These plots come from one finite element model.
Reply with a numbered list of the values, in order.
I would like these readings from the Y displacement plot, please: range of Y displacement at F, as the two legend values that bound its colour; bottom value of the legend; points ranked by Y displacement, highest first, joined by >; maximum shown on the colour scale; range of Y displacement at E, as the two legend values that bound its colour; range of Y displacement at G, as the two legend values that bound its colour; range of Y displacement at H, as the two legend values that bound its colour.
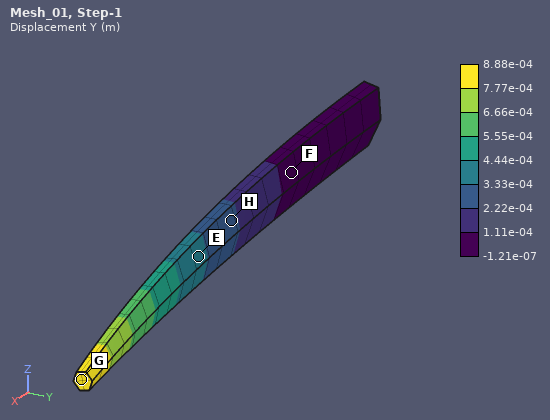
1. -1.21e-07 to 1.11e-04 m
2. -1.21e-07 m
3. G > E > H > F
4. 8.88e-04 m
5. 3.33e-04 to 4.44e-04 m
6. 7.77e-04 to 8.88e-04 m
7. 2.22e-04 to 3.33e-04 m
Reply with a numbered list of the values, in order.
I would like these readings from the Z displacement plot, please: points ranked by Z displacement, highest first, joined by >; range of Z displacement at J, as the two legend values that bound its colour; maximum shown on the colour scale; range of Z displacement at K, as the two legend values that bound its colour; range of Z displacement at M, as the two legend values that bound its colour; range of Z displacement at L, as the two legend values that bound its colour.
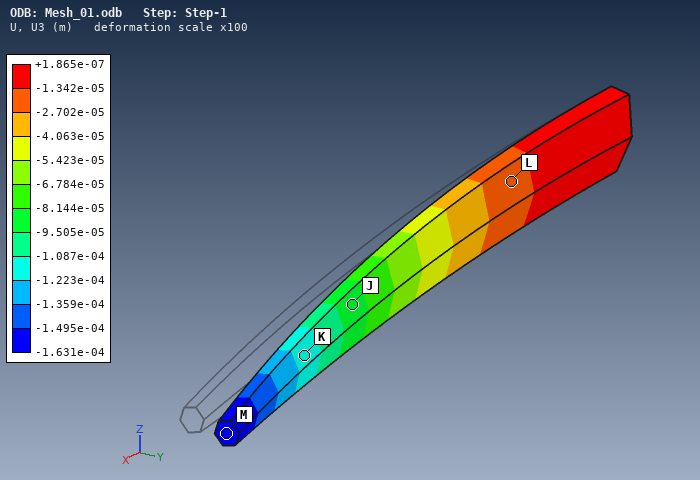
1. L > J > K > M
2. -9.505e-05 to -8.144e-05 m
3. +1.865e-07 m
4. -1.223e-04 to -1.087e-04 m
5. -1.631e-04 to -1.495e-04 m
6. -2.702e-05 to -1.342e-05 m
